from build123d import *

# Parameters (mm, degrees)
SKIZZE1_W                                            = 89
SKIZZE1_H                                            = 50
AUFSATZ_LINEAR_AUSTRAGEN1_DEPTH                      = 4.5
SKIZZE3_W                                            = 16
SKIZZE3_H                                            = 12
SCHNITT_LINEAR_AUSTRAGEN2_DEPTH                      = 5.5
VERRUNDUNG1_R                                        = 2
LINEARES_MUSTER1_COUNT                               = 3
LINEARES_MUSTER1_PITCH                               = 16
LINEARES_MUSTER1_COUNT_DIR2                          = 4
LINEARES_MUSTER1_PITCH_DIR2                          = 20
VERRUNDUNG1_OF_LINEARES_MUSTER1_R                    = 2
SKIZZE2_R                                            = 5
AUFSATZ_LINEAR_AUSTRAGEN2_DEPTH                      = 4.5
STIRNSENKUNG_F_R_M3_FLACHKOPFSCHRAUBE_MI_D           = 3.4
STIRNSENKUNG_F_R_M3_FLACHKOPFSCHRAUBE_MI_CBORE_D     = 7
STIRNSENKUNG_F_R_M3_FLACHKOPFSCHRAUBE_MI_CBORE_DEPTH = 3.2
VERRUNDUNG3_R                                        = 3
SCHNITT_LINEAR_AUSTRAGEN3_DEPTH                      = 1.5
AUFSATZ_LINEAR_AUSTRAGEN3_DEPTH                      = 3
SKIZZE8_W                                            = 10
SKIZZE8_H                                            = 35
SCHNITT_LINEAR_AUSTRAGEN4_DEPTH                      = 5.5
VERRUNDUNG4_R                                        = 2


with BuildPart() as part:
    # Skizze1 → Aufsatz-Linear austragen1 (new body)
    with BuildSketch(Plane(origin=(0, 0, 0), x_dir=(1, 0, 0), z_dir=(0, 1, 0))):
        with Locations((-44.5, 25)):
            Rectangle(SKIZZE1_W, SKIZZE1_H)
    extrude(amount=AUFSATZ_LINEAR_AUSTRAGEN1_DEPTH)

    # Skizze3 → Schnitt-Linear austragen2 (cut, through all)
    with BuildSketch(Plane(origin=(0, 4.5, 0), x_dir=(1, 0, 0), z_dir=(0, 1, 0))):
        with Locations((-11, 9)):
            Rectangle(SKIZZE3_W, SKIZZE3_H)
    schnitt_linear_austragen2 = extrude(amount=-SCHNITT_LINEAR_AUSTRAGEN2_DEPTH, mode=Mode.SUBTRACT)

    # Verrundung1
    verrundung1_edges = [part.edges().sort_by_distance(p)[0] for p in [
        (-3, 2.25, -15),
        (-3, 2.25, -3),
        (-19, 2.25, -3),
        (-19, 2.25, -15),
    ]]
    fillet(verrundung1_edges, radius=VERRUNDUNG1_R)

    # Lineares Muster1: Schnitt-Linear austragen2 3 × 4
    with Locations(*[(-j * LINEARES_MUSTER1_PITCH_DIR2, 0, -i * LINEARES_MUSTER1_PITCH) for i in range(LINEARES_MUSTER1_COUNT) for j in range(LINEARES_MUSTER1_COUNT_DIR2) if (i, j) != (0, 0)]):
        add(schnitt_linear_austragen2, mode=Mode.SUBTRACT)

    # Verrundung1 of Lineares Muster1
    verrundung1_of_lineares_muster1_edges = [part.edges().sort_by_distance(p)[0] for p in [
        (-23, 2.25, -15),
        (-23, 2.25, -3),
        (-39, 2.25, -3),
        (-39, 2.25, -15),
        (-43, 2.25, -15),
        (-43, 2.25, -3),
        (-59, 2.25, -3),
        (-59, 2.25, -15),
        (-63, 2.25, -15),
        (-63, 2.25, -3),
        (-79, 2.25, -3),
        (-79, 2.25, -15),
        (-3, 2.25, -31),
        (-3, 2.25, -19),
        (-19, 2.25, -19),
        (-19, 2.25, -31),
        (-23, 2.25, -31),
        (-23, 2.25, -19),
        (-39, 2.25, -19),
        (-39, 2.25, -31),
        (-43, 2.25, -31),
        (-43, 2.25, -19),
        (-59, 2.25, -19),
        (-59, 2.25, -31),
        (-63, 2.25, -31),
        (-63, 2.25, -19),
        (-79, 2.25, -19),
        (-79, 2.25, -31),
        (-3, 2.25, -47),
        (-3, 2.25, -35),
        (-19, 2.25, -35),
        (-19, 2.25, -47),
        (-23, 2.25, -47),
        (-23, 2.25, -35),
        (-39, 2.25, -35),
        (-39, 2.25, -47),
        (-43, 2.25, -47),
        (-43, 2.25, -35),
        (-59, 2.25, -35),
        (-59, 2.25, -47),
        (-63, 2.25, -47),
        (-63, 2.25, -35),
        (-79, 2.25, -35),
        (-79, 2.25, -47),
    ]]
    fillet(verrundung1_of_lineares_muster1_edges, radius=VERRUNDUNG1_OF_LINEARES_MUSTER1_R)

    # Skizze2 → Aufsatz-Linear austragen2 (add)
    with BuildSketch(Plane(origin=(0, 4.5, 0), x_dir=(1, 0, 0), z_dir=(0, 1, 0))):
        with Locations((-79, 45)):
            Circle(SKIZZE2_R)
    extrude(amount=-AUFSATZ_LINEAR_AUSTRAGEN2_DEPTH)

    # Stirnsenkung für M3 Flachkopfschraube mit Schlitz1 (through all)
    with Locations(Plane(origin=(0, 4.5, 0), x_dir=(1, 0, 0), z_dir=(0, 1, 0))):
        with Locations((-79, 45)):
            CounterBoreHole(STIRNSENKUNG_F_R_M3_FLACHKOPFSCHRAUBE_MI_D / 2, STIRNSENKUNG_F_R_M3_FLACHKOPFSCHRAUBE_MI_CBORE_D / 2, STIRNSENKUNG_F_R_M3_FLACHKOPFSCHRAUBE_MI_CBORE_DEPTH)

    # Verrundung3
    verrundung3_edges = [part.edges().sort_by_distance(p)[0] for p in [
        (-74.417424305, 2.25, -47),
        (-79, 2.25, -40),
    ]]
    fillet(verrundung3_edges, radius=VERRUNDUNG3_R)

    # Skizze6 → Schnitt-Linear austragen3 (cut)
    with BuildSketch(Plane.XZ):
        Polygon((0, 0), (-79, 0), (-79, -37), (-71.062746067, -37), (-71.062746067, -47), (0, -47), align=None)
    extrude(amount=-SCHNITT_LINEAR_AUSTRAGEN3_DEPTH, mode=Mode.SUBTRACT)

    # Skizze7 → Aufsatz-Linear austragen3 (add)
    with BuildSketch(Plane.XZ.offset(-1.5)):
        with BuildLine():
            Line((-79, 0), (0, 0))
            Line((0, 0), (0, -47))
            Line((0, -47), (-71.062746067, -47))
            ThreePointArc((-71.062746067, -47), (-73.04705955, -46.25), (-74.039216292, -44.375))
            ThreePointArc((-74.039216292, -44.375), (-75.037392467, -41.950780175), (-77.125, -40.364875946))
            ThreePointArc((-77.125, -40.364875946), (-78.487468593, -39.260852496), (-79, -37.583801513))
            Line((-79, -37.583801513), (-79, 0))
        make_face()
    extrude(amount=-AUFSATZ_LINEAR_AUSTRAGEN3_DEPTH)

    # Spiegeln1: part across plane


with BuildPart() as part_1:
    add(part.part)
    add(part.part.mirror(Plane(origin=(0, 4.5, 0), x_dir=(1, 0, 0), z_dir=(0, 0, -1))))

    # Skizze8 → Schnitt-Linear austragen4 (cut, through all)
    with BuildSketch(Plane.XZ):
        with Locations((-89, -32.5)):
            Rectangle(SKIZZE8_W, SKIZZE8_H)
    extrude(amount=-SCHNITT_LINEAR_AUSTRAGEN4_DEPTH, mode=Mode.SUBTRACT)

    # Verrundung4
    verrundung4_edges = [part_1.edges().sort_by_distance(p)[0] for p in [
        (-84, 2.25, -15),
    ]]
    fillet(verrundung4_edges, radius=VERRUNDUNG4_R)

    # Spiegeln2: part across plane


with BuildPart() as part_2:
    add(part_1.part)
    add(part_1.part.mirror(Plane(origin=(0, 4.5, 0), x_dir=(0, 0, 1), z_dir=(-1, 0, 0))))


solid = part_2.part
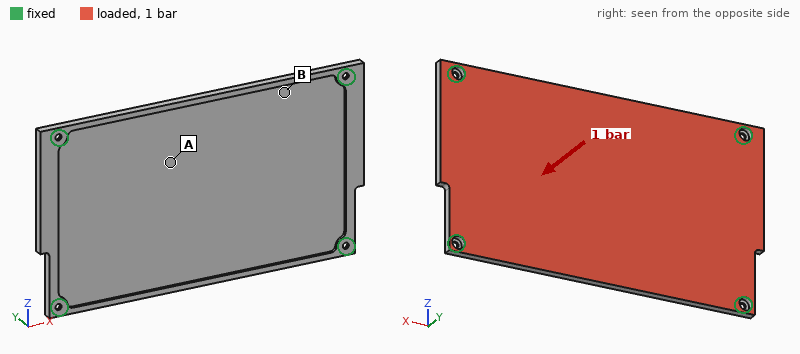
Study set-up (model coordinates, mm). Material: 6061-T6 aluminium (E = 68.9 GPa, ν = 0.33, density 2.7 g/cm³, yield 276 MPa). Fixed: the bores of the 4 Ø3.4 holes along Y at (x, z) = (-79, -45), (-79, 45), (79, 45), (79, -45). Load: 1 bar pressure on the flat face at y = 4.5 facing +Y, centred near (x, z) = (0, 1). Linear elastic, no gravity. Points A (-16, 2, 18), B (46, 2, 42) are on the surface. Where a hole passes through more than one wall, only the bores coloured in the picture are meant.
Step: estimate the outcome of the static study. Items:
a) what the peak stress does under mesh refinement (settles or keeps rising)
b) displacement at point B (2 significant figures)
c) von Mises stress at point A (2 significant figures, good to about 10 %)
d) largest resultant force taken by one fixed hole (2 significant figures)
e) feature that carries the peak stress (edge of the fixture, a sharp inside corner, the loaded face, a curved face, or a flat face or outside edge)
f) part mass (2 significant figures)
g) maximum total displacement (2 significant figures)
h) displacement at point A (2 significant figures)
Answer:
keeps rising
0.69 mm
49 MPa
2.2 kN
edge of the fixture
150 g
1.4 mm
1.3 mm
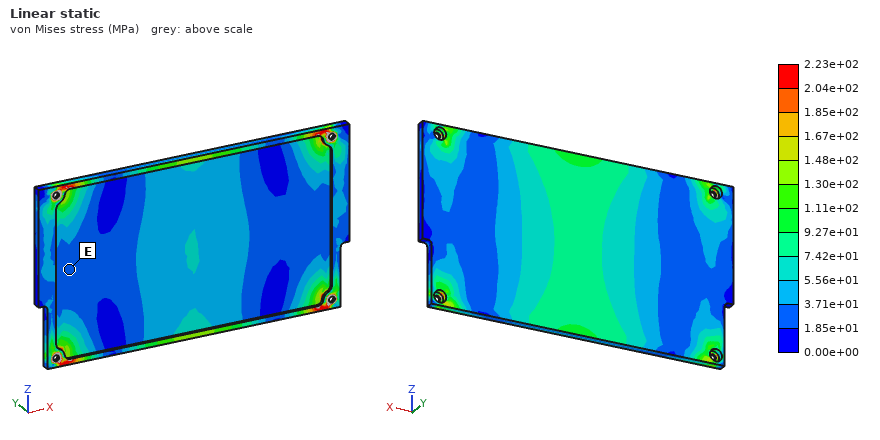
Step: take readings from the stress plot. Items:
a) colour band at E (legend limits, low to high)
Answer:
1.85e+01 to 3.71e+01 MPa
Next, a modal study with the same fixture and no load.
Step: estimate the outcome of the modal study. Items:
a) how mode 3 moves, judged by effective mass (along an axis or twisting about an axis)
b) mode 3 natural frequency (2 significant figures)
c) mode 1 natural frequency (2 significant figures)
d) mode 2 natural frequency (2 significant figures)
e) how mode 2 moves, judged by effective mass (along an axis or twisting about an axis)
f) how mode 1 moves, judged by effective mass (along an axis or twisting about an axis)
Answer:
twisting about Z
1300 Hz
530 Hz
900 Hz
twisting about X
along Y
